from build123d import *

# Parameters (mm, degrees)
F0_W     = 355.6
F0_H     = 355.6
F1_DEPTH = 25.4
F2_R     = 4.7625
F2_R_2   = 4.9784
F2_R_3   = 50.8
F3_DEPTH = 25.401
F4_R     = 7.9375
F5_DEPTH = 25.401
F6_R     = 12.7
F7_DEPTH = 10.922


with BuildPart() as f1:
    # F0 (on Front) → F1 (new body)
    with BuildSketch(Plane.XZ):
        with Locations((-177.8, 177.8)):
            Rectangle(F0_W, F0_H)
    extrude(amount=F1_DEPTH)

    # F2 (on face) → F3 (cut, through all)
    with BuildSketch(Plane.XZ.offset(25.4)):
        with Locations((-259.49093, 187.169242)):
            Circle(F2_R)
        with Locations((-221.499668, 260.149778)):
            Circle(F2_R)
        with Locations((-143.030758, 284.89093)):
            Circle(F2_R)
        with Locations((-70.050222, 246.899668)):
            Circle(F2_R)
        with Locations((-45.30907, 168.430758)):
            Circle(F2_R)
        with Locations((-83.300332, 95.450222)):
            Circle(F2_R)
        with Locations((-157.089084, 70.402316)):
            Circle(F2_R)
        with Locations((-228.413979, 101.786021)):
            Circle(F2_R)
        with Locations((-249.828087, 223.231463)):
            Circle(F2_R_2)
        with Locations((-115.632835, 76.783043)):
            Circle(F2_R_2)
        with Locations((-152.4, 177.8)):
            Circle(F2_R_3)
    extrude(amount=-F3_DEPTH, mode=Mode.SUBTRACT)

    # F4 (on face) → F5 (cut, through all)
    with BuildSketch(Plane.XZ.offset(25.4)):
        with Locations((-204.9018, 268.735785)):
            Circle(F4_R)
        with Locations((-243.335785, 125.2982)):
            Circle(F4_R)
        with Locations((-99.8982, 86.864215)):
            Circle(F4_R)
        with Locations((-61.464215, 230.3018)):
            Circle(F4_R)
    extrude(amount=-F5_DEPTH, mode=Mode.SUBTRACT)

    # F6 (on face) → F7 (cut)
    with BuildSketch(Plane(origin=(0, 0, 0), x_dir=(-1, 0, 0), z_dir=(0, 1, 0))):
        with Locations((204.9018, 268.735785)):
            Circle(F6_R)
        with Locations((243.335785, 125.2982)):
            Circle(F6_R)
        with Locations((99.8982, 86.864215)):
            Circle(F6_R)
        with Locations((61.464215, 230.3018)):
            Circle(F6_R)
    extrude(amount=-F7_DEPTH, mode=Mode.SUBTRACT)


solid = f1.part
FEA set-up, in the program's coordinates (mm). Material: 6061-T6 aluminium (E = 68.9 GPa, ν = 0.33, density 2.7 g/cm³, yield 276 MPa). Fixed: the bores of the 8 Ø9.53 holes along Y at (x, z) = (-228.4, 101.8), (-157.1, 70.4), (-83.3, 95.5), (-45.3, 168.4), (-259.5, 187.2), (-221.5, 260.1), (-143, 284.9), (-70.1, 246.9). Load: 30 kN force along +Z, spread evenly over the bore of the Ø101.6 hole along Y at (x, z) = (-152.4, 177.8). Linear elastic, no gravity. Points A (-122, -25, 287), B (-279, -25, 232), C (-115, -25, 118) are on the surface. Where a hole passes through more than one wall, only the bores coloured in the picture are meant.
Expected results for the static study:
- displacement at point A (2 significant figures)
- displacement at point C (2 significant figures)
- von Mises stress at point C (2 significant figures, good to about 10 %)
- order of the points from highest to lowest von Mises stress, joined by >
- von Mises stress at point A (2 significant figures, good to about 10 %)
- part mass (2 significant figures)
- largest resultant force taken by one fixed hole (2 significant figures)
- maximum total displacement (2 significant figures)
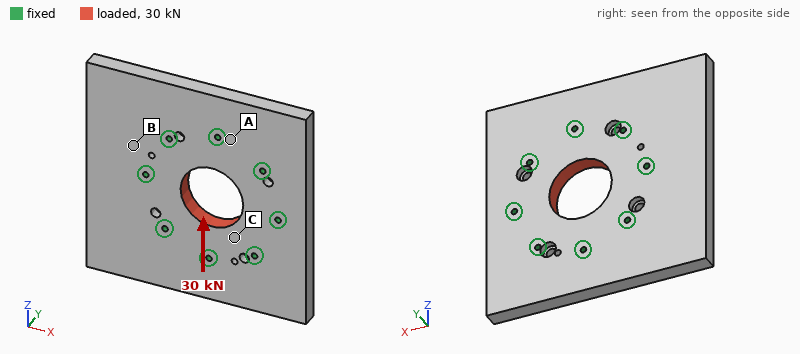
1.2 µm
2.8 µm
2.9 MPa
C > A > B
1.7 MPa
8.0 kg
5.7 kN
4.3 µm
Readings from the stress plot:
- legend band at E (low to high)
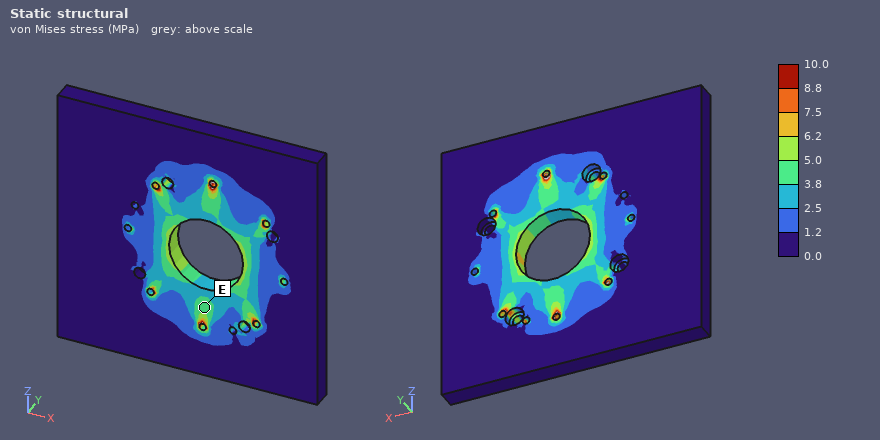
3.8 to 5.0 MPa
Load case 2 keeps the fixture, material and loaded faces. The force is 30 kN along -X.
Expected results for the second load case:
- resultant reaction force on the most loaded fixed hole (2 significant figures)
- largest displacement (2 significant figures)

5.8 kN
4.3 µm
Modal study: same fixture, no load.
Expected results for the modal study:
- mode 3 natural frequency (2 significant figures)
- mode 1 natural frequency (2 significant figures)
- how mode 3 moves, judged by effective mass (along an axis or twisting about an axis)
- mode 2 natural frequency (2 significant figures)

1700 Hz
1100 Hz
along Y
1100 Hz
